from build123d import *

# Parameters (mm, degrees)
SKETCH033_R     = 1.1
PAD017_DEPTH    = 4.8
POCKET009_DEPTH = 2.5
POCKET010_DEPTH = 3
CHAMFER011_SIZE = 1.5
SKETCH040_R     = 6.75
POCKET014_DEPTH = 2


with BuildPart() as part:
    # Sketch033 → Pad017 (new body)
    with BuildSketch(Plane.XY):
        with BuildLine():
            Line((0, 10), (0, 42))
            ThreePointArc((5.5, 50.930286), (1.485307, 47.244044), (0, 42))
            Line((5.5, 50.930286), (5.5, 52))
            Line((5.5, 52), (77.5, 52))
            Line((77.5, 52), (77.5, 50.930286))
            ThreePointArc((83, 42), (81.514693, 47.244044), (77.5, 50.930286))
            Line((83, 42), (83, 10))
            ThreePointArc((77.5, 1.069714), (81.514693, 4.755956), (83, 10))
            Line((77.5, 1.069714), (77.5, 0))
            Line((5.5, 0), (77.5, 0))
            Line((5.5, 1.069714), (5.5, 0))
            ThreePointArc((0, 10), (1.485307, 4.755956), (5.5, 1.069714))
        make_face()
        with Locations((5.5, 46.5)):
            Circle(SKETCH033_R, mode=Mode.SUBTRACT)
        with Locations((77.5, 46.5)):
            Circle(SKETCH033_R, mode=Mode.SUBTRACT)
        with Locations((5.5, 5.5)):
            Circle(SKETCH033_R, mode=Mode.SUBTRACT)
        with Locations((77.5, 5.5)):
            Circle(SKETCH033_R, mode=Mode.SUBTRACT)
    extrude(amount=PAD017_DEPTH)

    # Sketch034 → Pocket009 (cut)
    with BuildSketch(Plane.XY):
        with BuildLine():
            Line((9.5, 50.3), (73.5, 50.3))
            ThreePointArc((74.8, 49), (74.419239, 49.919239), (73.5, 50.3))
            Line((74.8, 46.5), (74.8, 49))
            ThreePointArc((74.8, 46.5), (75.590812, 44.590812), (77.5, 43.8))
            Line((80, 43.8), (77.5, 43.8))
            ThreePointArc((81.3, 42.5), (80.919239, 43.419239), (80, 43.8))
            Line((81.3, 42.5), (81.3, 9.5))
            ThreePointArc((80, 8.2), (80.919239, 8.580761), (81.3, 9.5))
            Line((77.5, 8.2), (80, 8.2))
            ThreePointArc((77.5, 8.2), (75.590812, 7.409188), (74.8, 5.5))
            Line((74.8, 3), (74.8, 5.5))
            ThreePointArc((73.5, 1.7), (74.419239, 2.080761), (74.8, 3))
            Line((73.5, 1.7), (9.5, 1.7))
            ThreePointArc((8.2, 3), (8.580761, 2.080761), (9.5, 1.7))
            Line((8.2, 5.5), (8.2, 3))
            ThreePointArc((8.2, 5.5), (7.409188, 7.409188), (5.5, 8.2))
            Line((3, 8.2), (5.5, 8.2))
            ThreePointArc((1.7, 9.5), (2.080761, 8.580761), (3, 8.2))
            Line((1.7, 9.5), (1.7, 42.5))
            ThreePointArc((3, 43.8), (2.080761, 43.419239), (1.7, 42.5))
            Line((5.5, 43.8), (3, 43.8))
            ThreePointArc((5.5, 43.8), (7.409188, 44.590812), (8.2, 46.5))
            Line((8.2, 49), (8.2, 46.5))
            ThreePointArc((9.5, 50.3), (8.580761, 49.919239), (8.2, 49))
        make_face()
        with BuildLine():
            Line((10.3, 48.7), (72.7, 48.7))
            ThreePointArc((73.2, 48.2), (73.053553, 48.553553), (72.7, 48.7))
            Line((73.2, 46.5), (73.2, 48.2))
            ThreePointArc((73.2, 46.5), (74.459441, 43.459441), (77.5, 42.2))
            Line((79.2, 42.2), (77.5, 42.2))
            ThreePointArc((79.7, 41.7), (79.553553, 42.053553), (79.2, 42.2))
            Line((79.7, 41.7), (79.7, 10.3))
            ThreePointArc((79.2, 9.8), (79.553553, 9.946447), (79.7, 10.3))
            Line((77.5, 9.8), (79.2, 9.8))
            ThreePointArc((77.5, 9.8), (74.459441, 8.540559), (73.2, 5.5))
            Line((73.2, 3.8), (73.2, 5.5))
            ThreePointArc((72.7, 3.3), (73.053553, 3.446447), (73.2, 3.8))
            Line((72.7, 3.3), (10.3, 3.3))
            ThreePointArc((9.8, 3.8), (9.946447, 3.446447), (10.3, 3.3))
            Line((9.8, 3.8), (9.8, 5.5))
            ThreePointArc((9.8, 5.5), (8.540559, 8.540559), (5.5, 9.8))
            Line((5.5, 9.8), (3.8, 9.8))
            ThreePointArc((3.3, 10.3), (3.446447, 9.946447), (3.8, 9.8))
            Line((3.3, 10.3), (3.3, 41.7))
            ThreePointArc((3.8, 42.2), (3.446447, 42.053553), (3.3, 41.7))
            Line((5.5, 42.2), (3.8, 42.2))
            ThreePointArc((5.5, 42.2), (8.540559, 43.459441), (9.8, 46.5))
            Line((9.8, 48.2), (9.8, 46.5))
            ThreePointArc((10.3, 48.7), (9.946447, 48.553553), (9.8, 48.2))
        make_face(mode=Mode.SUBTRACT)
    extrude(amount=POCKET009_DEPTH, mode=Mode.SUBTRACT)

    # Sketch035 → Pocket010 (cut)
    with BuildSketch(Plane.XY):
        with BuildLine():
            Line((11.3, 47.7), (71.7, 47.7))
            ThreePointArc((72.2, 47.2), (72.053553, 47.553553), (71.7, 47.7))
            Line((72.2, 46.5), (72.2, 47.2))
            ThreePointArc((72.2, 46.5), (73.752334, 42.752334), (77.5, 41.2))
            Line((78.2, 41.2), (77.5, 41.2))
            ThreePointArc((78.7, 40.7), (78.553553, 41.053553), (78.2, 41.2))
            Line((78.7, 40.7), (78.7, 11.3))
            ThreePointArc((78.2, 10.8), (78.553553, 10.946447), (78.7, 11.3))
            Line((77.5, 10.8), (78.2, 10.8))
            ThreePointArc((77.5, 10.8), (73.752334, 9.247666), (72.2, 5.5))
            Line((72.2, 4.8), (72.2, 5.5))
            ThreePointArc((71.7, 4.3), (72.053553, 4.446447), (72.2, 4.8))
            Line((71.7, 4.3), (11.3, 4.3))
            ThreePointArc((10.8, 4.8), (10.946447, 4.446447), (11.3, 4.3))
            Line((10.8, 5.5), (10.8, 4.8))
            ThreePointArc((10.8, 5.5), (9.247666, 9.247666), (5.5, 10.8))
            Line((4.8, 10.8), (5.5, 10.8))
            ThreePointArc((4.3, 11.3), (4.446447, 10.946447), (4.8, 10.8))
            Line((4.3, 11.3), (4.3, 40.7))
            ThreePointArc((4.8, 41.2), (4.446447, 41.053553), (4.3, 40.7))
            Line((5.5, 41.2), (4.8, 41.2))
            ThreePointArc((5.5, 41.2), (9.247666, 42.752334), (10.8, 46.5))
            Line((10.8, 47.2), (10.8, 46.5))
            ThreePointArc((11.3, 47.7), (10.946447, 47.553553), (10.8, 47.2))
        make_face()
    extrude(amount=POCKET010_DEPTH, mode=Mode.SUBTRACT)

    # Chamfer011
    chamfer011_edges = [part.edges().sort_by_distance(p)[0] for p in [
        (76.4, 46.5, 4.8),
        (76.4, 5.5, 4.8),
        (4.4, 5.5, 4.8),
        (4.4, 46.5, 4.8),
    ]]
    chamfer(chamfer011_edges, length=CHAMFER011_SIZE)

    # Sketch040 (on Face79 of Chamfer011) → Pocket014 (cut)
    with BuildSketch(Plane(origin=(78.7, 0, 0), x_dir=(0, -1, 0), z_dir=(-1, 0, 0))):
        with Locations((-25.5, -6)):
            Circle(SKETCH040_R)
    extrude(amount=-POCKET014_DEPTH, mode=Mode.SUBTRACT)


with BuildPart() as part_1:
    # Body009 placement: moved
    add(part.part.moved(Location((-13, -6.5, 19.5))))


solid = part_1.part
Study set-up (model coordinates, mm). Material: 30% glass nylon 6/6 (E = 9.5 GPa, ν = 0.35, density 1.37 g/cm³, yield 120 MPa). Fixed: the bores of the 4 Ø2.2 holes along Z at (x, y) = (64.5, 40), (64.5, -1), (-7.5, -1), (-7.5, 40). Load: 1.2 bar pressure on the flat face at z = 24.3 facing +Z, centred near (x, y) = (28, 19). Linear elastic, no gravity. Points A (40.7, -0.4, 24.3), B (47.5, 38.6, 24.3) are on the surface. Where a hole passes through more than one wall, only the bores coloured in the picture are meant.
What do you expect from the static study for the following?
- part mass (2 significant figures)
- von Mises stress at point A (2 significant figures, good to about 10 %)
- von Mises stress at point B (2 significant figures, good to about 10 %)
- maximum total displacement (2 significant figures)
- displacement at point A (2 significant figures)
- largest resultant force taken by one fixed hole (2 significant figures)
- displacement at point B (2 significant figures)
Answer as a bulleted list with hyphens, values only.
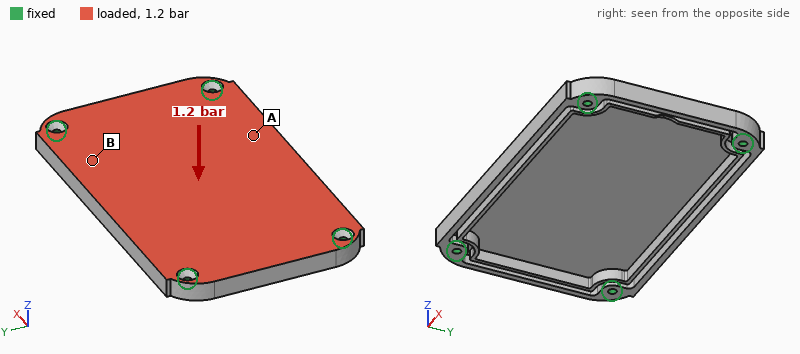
- 14 g
- 17 MPa
- 11 MPa
- 1.0 mm
- 0.55 mm
- 190 N
- 0.41 mm
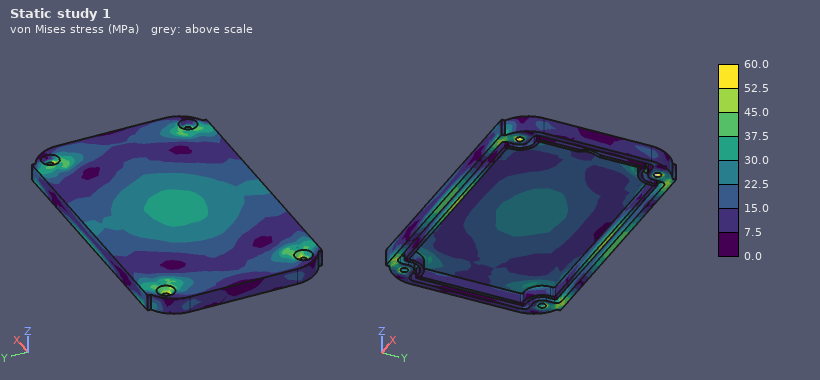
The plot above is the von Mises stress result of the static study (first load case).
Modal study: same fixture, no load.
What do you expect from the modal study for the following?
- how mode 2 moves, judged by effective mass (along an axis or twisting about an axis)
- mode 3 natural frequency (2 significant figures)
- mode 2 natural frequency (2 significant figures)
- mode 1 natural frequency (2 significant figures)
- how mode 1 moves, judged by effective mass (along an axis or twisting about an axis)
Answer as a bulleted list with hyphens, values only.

- twisting about X
- 2800 Hz
- 2000 Hz
- 1300 Hz
- along Z
